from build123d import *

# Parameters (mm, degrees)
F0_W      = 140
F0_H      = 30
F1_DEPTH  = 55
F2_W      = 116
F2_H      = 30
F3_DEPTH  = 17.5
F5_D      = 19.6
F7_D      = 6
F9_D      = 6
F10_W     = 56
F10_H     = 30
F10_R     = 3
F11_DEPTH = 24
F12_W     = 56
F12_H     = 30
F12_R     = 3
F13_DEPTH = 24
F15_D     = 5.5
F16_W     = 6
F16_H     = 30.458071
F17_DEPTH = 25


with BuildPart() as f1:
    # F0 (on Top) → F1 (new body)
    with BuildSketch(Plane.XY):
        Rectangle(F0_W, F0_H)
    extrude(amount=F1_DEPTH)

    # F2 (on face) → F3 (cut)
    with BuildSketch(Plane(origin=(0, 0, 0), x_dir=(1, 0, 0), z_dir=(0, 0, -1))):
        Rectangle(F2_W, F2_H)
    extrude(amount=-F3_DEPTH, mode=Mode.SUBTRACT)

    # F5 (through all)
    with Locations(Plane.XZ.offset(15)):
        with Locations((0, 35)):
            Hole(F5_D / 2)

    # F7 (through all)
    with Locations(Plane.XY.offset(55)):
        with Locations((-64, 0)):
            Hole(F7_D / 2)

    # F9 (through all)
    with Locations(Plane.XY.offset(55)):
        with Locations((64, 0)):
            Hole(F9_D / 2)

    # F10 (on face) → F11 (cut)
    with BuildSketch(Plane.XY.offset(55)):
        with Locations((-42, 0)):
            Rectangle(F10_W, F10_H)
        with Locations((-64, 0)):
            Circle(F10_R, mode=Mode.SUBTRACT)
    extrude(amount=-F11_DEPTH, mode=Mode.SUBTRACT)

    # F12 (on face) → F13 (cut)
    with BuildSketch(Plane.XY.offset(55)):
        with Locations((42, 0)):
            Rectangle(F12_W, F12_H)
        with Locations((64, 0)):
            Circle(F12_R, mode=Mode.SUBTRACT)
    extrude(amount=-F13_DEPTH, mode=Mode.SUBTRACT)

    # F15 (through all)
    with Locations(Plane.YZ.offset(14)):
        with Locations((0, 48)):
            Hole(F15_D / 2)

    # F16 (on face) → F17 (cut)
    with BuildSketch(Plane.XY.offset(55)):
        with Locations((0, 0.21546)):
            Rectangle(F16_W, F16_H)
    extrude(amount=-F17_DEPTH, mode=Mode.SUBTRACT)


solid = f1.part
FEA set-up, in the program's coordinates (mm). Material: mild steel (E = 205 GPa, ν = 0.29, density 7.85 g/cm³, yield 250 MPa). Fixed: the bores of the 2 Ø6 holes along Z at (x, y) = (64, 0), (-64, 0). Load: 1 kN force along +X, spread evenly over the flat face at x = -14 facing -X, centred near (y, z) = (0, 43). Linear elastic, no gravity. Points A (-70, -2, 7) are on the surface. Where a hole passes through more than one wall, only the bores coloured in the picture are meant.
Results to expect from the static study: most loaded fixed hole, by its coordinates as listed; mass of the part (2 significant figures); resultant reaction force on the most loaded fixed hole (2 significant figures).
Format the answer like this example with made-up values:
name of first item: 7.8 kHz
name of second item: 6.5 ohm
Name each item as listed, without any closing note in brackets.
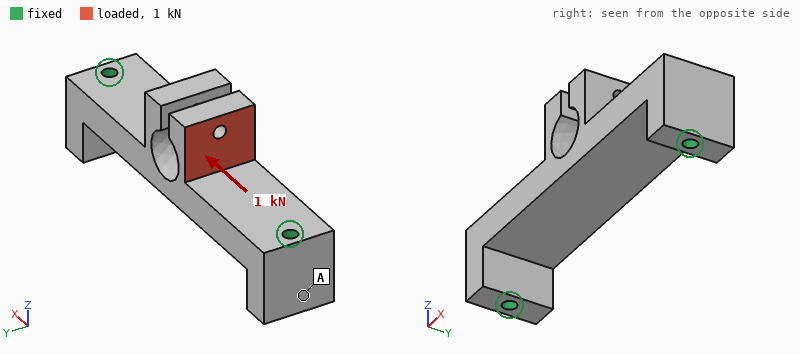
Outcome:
most loaded fixed hole, by its coordinates as listed: (-64, 0)
mass of the part: 600 g
resultant reaction force on the most loaded fixed hole: 1.0 kN
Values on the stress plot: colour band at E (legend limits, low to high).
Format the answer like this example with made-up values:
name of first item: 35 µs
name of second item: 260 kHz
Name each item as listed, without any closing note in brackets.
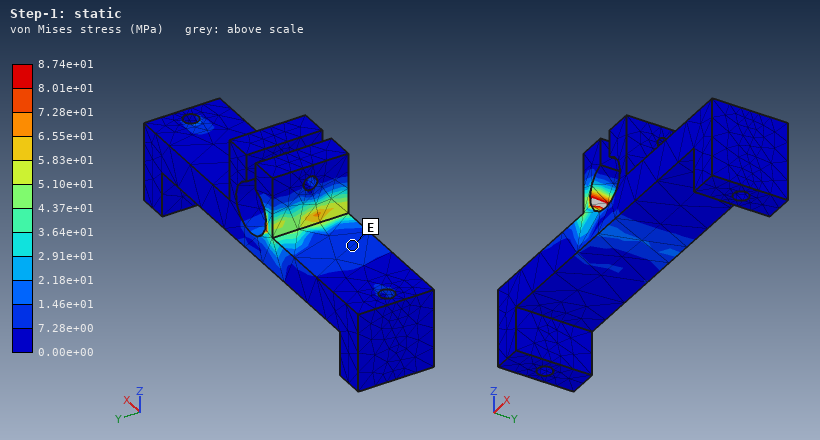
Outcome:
colour band at E: 7.28e+00 to 1.46e+01 MPa
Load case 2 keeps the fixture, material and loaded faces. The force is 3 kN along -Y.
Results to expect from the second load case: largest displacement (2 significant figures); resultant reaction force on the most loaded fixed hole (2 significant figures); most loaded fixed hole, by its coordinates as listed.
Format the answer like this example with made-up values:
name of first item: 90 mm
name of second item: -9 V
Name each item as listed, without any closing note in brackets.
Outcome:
largest displacement: 63 µm
resultant reaction force on the most loaded fixed hole: 1.9 kN
most loaded fixed hole, by its coordinates as listed: (-64, 0)
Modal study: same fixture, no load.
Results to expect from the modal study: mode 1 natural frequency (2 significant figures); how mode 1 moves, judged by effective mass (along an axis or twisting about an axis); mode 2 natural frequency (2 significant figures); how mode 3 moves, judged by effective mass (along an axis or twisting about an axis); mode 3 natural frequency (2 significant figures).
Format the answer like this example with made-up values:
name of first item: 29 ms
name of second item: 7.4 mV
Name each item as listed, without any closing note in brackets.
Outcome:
mode 1 natural frequency: 2700 Hz
how mode 1 moves, judged by effective mass: along Z
mode 2 natural frequency: 3700 Hz
how mode 3 moves, judged by effective mass: along Y
mode 3 natural frequency: 3900 Hz
